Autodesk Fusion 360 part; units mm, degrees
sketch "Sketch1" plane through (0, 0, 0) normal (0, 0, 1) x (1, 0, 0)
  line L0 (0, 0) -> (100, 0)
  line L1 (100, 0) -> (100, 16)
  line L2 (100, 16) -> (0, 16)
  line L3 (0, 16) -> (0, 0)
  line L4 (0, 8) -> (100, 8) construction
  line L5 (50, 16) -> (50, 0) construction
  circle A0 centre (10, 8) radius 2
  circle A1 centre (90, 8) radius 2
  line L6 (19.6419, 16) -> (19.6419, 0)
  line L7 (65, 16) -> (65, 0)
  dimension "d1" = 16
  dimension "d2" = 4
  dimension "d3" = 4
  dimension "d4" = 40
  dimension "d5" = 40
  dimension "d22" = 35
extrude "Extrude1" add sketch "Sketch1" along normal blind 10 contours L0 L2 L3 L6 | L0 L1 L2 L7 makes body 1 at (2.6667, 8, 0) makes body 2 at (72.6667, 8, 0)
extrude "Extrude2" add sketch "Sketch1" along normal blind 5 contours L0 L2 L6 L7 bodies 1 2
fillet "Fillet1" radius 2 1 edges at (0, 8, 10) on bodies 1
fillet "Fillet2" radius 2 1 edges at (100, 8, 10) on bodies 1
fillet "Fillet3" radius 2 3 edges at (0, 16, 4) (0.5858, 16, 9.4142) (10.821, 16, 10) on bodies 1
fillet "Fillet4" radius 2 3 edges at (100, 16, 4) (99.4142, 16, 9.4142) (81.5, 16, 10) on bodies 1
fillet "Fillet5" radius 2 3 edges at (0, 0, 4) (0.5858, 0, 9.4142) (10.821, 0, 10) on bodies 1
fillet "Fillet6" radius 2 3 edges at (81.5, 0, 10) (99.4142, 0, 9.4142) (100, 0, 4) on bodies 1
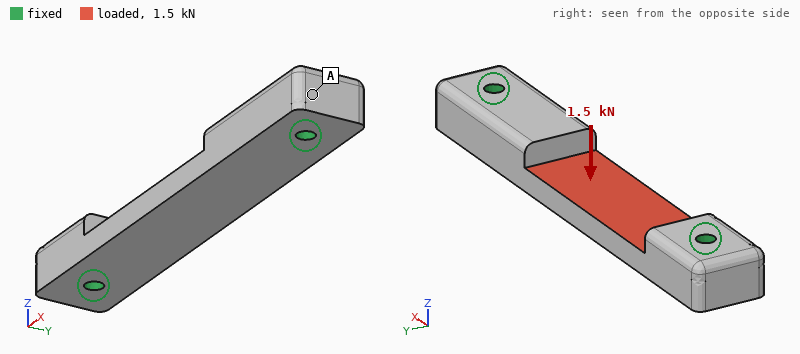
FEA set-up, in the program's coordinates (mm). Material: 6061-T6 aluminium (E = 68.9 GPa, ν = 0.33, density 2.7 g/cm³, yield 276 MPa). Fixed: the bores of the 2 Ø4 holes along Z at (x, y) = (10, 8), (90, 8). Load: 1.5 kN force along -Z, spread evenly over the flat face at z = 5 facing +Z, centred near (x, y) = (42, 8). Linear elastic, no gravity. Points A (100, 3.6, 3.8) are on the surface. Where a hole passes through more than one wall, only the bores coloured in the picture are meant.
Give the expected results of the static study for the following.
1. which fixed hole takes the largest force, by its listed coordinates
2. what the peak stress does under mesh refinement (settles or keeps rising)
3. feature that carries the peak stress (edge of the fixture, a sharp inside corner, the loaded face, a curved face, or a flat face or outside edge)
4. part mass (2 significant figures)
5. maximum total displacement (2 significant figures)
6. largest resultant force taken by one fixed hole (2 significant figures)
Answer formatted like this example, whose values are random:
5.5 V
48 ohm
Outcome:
(10, 8)
keeps rising
edge of the fixture
32 g
98 µm
1.1 kN
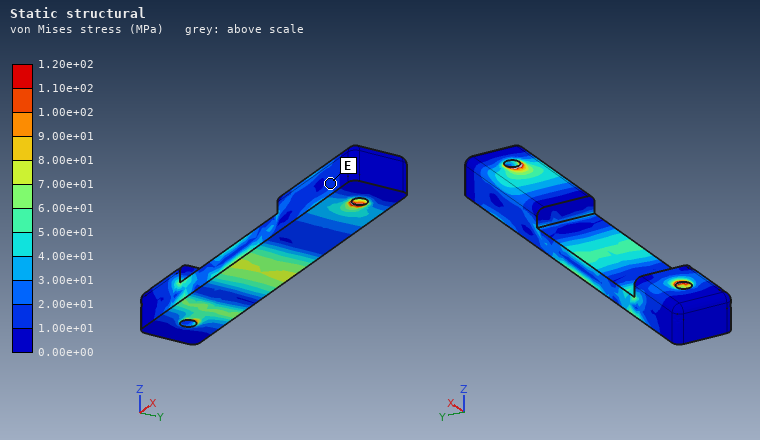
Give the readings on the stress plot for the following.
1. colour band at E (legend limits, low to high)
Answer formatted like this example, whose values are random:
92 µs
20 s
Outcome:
1.00e+01 to 2.00e+01 MPa
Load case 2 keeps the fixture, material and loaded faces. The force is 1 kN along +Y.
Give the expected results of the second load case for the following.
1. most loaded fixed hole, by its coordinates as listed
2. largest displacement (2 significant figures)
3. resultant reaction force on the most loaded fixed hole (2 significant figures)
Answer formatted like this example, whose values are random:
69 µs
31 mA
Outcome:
(10, 8)
32 µm
610 N
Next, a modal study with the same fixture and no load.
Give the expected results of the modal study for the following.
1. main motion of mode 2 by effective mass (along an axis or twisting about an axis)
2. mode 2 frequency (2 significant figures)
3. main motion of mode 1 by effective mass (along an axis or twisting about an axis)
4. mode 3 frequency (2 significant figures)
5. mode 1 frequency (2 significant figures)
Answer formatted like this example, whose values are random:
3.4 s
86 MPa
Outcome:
along Y
8800 Hz
along Z
14 kHz
6600 Hz
